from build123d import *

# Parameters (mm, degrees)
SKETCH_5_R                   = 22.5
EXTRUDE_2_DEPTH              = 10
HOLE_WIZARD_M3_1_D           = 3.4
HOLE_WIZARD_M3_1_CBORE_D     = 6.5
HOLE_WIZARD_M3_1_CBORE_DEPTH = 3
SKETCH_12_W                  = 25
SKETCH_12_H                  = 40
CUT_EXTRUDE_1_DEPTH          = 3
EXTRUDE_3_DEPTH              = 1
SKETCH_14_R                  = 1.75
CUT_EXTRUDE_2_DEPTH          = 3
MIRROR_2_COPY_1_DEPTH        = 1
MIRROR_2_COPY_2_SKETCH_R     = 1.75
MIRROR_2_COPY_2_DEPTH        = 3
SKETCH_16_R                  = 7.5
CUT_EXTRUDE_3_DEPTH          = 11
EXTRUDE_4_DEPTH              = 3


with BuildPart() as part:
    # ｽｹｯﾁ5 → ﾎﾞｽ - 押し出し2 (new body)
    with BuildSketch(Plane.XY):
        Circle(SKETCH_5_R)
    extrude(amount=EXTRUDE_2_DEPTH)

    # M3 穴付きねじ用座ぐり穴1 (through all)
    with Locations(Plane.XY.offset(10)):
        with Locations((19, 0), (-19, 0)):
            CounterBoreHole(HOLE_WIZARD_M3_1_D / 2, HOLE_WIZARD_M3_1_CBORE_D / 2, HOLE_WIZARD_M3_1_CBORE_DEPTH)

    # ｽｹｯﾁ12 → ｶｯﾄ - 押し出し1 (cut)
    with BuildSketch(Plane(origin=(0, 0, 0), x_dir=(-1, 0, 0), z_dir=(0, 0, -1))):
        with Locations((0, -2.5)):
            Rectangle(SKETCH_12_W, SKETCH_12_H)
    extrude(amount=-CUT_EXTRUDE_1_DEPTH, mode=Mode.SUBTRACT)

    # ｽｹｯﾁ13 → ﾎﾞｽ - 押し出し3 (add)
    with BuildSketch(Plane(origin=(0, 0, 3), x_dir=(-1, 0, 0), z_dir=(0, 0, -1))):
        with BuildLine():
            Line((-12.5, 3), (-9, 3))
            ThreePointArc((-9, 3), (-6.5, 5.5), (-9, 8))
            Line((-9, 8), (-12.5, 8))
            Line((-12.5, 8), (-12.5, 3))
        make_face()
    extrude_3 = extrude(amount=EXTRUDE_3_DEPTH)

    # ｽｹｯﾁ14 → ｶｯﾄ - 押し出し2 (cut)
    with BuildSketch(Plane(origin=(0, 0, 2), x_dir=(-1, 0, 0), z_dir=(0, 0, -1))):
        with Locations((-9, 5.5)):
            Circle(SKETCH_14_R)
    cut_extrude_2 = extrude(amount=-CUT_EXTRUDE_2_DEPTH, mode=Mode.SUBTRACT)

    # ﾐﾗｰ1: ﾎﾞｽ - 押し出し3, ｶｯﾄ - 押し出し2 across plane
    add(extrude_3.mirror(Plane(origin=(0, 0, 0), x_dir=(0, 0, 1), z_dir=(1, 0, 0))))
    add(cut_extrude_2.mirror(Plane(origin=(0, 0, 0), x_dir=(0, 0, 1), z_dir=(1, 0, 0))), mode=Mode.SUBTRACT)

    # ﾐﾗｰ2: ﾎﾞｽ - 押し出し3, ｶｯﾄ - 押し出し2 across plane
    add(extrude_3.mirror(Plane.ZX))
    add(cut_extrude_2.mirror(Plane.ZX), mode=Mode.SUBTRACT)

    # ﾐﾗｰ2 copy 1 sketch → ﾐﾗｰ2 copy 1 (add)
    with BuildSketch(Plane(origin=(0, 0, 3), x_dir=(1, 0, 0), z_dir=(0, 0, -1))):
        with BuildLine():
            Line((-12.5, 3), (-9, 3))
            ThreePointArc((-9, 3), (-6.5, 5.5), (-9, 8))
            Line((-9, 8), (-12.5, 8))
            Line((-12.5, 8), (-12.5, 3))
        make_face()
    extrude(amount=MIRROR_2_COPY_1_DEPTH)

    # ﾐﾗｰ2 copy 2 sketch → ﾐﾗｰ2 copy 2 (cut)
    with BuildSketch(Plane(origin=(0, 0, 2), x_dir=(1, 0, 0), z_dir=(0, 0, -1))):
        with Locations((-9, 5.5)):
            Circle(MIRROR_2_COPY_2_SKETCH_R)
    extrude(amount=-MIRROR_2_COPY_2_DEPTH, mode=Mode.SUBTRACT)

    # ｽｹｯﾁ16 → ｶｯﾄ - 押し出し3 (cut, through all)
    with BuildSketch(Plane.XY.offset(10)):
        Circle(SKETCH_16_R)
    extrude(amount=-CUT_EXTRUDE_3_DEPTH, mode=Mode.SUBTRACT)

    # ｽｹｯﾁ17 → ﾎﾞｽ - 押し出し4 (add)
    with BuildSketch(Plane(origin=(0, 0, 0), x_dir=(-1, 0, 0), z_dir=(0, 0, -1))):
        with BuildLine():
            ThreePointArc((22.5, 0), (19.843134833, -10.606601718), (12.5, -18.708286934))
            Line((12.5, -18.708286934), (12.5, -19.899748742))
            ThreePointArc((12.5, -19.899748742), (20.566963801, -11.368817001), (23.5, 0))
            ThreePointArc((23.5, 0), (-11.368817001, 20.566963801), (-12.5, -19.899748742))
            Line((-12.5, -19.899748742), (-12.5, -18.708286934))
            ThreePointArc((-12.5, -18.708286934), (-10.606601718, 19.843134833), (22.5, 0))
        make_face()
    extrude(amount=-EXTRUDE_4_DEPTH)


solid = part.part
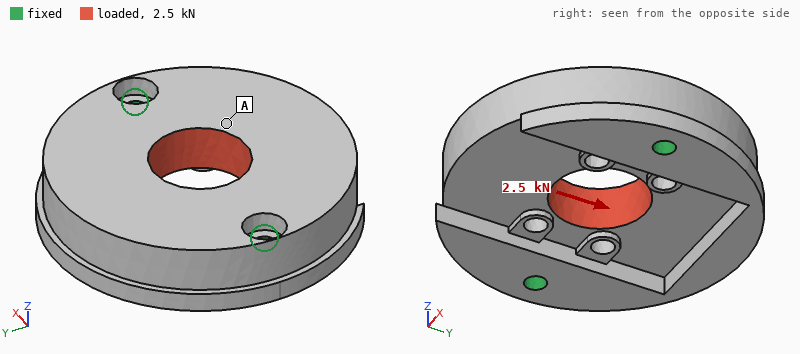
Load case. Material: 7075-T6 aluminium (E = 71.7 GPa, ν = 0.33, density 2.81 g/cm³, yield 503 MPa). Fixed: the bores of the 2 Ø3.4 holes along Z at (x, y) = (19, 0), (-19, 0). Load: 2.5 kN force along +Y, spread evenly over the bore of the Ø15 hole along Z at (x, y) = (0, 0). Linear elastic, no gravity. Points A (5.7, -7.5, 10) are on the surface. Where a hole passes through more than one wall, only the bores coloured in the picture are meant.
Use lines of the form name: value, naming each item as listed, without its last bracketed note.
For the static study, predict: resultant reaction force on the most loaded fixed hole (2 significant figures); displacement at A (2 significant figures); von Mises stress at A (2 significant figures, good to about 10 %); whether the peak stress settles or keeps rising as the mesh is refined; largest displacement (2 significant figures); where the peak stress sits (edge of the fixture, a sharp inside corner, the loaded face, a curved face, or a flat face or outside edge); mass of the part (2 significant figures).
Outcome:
resultant reaction force on the most loaded fixed hole: 1.3 kN
displacement at A: 7.6 µm
von Mises stress at A: 7.3 MPa
whether the peak stress settles or keeps rising as the mesh is refined: keeps rising
largest displacement: 13 µm
where the peak stress sits: edge of the fixture
mass of the part: 33 g
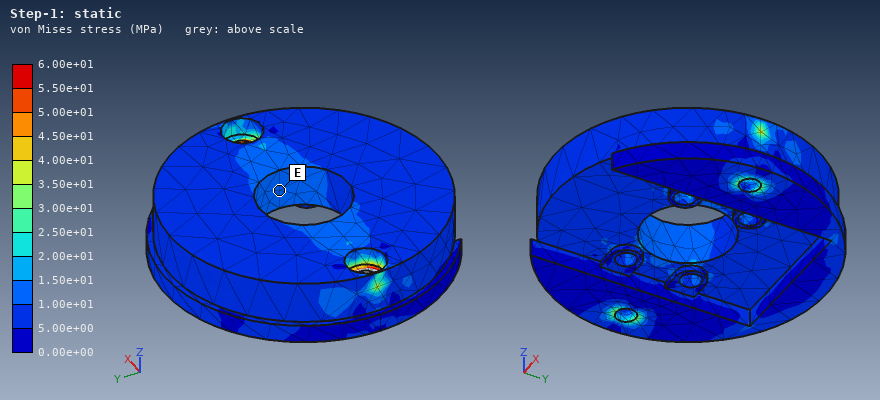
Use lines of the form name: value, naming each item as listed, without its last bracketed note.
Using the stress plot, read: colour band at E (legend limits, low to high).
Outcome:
colour band at E: 1.00e+01 to 1.50e+01 MPa
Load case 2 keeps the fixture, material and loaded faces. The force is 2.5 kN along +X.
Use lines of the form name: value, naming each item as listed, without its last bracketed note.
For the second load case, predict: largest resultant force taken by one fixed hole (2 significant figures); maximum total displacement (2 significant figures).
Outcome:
largest resultant force taken by one fixed hole: 1.3 kN
maximum total displacement: 4.2 µm
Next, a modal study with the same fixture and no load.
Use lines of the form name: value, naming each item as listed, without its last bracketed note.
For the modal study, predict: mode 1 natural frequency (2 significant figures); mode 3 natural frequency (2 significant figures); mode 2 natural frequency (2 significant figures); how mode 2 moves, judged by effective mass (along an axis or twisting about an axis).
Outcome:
mode 1 natural frequency: 8300 Hz
mode 3 natural frequency: 20 kHz
mode 2 natural frequency: 12 kHz
how mode 2 moves, judged by effective mass: along Z
